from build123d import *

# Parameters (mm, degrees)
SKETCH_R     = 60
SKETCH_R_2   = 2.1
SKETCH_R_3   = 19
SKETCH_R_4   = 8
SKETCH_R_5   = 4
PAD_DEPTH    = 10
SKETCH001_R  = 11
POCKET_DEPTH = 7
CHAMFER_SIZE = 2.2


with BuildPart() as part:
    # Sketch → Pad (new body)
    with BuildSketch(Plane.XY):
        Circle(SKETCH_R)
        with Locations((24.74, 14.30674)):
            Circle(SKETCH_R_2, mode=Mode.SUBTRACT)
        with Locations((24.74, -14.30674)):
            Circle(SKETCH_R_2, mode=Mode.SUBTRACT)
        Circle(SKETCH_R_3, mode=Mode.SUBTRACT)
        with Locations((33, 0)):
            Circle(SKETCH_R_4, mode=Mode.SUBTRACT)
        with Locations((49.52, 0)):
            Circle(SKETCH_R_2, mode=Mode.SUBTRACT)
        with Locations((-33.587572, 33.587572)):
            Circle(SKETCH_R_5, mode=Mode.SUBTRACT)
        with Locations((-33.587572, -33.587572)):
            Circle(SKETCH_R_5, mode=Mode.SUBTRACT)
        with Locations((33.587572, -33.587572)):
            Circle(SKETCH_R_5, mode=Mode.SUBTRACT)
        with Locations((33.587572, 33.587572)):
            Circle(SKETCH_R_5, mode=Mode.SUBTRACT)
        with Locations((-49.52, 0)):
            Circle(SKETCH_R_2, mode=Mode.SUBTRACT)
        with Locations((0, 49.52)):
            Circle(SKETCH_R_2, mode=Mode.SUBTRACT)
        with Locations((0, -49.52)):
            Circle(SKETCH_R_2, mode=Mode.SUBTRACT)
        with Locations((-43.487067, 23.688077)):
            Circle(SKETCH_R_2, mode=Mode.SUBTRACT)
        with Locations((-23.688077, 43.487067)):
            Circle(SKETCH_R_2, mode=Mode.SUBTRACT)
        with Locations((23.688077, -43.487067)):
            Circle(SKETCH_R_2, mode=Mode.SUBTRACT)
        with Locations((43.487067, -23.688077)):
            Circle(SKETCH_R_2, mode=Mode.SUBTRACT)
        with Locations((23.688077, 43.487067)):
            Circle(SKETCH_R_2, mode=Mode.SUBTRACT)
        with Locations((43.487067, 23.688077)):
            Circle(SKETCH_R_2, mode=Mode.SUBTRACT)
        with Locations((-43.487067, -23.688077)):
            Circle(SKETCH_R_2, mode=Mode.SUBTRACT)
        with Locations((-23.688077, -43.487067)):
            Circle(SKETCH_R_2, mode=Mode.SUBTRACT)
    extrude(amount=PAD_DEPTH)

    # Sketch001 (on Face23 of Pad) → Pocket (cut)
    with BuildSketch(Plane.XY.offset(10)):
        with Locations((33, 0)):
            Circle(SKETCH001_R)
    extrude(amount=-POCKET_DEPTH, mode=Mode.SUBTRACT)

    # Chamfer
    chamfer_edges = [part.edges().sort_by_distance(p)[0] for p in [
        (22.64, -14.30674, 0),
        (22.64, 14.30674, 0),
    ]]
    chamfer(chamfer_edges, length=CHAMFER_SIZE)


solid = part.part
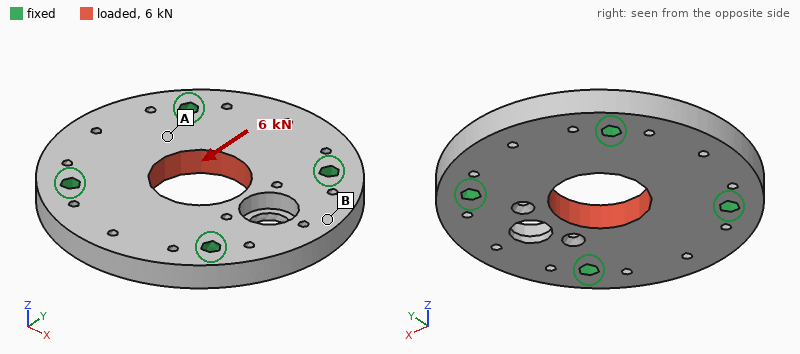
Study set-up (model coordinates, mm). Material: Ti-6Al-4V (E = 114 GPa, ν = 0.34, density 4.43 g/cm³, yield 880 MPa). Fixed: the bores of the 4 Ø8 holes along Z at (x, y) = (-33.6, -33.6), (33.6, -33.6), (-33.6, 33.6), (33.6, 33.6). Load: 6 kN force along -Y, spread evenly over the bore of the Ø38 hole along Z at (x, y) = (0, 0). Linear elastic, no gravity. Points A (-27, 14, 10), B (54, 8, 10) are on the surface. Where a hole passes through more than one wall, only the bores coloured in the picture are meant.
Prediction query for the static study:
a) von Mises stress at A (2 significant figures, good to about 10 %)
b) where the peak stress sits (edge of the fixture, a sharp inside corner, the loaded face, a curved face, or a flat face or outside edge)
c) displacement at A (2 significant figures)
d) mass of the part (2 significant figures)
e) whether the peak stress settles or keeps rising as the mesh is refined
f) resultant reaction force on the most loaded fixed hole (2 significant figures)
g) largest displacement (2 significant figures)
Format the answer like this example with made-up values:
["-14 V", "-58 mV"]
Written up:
["5.4 MPa", "edge of the fixture", "0.97 µm", "420 g", "keeps rising", "1.7 kN", "2.8 µm"]
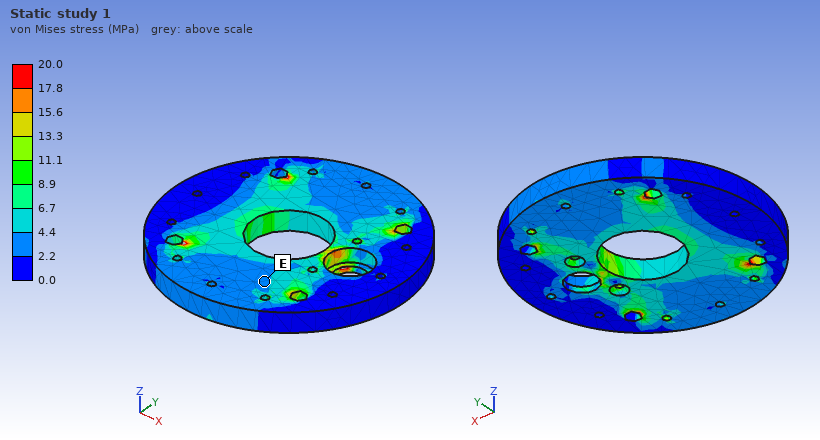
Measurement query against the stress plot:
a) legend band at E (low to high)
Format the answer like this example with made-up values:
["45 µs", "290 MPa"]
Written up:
["2.2 to 4.4 MPa"]
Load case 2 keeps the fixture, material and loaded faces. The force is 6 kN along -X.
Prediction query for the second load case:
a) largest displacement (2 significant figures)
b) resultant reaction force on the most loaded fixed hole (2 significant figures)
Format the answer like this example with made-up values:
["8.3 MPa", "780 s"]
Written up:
["5.2 µm", "1.6 kN"]
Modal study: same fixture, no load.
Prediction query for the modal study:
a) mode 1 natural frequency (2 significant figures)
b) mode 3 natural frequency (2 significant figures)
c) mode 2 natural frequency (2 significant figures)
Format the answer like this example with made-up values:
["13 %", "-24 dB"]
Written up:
["7600 Hz", "8100 Hz", "8100 Hz"]
